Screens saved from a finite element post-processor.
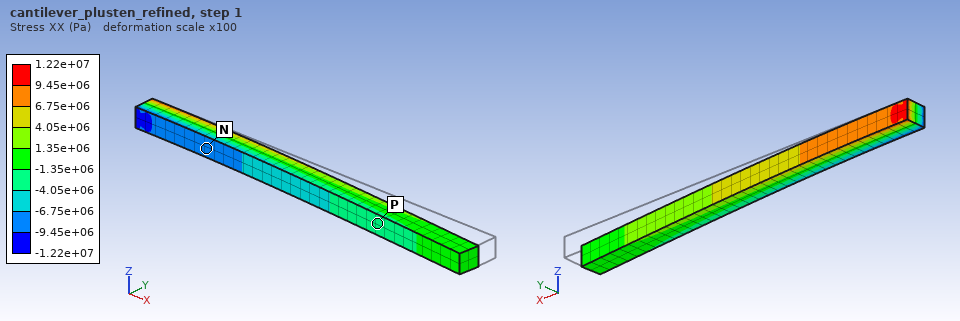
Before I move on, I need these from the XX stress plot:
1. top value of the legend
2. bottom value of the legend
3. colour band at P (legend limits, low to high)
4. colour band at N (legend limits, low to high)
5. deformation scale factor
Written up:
1.22e+07 Pa
-1.22e+07 Pa
-4.05e+06 to -1.35e+06 Pa
-9.45e+06 to -6.75e+06 Pa
100
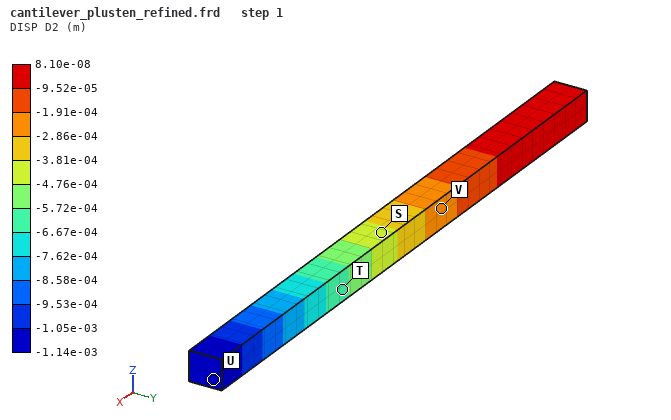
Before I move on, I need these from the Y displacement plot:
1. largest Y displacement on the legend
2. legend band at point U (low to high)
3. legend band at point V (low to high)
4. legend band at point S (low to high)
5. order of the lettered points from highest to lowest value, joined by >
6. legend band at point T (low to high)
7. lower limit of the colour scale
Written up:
8.10e-08 m
-1.14e-03 to -1.05e-03 m
-2.86e-04 to -1.91e-04 m
-4.76e-04 to -3.81e-04 m
V > S > T > U
-6.67e-04 to -5.72e-04 m
-1.14e-03 m
